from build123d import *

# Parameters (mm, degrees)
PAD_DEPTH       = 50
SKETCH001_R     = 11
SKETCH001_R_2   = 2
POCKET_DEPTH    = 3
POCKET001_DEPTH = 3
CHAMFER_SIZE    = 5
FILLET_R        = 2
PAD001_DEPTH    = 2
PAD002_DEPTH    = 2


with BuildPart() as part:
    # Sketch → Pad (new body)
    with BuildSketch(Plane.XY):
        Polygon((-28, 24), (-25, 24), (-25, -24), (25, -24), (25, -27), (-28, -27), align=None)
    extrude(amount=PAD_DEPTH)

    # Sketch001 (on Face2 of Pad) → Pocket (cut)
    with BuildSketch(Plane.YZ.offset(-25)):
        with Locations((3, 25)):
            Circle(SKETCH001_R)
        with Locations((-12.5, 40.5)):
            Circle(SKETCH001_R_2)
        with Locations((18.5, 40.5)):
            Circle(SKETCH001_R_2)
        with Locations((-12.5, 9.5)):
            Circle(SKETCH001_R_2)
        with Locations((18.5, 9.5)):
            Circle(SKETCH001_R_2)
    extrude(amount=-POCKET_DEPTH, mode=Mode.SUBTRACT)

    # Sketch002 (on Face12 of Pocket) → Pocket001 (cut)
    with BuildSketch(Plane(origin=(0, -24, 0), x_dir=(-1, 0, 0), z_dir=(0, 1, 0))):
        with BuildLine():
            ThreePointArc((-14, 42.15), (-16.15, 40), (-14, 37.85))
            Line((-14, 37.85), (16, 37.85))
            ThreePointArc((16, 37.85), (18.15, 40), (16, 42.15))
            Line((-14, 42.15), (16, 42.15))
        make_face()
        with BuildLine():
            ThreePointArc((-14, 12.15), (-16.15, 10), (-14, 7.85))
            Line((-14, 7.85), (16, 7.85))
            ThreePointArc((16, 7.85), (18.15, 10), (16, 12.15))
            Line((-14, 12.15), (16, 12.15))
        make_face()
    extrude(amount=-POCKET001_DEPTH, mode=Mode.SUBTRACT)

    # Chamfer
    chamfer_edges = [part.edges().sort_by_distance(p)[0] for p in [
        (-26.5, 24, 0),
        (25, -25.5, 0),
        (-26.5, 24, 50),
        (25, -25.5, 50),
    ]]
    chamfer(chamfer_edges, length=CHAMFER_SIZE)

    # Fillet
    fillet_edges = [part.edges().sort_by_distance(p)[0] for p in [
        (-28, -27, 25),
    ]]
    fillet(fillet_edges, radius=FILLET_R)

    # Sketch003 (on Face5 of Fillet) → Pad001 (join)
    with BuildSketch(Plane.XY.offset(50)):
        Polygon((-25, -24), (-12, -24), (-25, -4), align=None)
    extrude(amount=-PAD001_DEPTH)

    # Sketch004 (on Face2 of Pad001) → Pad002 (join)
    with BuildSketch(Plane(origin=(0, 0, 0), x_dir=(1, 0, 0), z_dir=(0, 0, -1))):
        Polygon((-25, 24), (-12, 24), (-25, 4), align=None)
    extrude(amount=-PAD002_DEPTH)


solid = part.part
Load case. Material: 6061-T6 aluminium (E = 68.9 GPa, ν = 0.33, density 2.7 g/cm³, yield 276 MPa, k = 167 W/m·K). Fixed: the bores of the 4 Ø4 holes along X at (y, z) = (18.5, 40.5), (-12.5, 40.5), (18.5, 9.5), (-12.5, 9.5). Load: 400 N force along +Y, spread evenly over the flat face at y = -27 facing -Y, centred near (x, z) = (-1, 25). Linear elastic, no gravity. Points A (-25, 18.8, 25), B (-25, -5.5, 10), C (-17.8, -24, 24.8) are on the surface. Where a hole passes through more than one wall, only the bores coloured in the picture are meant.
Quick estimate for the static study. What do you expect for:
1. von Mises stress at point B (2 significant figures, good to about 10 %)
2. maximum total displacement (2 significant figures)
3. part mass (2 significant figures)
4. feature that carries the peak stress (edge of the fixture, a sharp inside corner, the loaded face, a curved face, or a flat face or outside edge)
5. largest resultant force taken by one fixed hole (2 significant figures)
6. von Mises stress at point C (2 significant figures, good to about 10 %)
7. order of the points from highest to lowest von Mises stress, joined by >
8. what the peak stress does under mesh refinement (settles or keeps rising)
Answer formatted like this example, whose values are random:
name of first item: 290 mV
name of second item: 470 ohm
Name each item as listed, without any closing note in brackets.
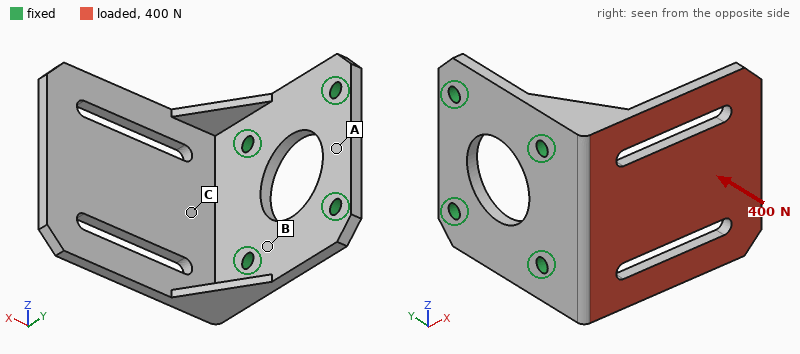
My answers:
von Mises stress at point B: 33 MPa
maximum total displacement: 1.0 mm
part mass: 36 g
feature that carries the peak stress: edge of the fixture
largest resultant force taken by one fixed hole: 210 N
von Mises stress at point C: 60 MPa
order of the points from highest to lowest von Mises stress, joined by >: C > B > A
what the peak stress does under mesh refinement: keeps rising
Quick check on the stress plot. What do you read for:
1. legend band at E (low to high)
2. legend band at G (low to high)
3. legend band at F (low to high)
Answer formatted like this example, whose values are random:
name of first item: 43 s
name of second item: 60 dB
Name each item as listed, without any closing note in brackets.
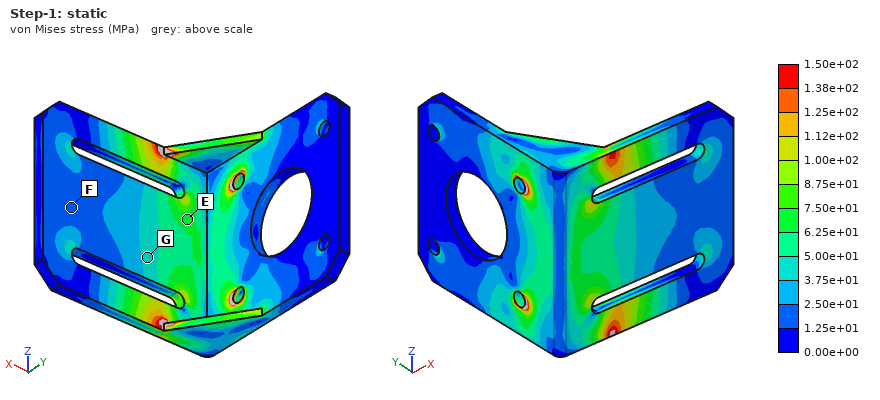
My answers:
legend band at E: 6.25e+01 to 7.50e+01 MPa
legend band at G: 3.75e+01 to 5.00e+01 MPa
legend band at F: 1.25e+01 to 2.50e+01 MPa
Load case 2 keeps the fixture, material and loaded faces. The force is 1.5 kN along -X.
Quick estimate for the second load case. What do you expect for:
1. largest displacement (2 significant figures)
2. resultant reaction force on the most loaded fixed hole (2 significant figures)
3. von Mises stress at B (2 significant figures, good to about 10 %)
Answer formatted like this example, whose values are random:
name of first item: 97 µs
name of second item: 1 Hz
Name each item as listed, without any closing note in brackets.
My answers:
largest displacement: 0.78 mm
resultant reaction force on the most loaded fixed hole: 860 N
von Mises stress at B: 40 MPa
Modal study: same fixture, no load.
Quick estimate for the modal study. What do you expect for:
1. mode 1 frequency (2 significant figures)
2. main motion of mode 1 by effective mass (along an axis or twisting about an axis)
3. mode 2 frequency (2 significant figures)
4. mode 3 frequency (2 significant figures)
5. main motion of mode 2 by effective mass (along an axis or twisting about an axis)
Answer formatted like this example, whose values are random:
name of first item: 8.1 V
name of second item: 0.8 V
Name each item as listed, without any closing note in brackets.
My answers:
mode 1 frequency: 920 Hz
main motion of mode 1 by effective mass: along Y
mode 2 frequency: 2100 Hz
mode 3 frequency: 3200 Hz
main motion of mode 2 by effective mass: along Z
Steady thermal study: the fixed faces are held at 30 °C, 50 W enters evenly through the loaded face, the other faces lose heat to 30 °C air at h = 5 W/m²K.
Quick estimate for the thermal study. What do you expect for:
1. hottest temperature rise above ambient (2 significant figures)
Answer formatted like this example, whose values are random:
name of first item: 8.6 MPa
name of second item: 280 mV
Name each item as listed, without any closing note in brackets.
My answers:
hottest temperature rise above ambient: 79 K
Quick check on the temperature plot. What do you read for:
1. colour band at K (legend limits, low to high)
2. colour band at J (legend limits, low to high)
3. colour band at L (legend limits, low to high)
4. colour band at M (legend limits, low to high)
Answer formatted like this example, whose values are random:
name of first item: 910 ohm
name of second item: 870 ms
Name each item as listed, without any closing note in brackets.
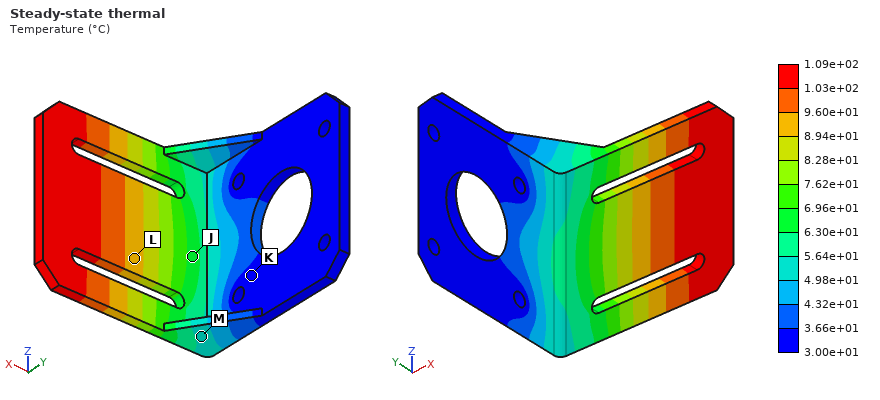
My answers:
colour band at K: 3.00e+01 to 3.66e+01 °C
colour band at J: 6.30e+01 to 6.96e+01 °C
colour band at L: 8.94e+01 to 9.60e+01 °C
colour band at M: 4.98e+01 to 5.64e+01 °C
